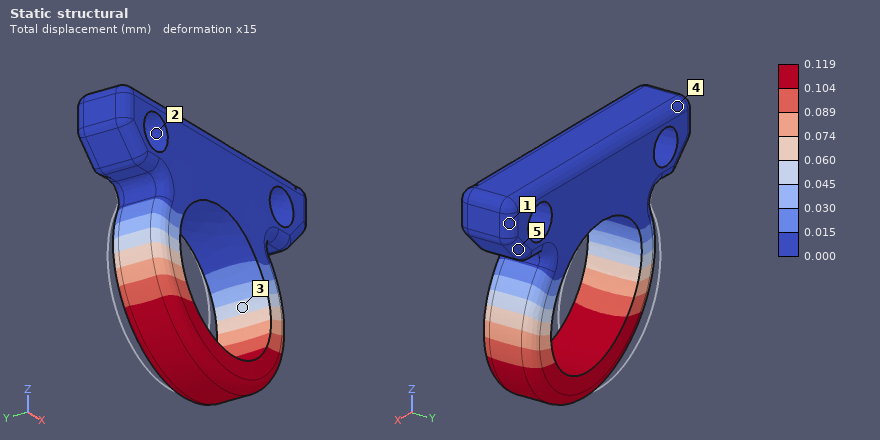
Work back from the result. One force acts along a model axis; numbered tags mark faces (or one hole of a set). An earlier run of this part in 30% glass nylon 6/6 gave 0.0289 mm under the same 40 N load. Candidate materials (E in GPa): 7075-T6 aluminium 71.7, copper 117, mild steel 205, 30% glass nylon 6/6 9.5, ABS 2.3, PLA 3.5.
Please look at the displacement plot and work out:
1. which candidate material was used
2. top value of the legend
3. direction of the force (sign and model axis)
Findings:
ABS
0.119 mm
+X
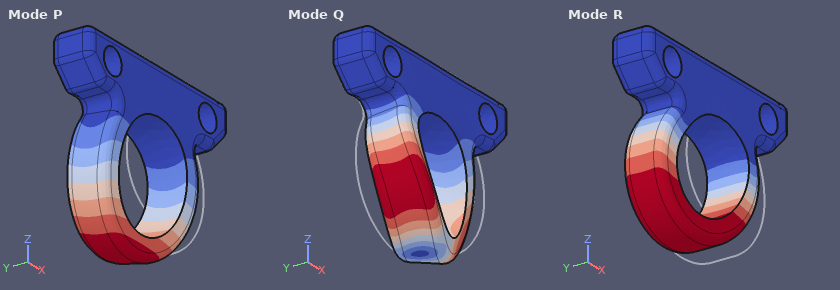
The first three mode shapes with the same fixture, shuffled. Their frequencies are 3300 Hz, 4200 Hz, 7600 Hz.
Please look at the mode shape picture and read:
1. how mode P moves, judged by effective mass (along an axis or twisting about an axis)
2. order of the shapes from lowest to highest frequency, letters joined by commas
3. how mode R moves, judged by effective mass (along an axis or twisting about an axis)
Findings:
along Y
P, R, Q
along X
